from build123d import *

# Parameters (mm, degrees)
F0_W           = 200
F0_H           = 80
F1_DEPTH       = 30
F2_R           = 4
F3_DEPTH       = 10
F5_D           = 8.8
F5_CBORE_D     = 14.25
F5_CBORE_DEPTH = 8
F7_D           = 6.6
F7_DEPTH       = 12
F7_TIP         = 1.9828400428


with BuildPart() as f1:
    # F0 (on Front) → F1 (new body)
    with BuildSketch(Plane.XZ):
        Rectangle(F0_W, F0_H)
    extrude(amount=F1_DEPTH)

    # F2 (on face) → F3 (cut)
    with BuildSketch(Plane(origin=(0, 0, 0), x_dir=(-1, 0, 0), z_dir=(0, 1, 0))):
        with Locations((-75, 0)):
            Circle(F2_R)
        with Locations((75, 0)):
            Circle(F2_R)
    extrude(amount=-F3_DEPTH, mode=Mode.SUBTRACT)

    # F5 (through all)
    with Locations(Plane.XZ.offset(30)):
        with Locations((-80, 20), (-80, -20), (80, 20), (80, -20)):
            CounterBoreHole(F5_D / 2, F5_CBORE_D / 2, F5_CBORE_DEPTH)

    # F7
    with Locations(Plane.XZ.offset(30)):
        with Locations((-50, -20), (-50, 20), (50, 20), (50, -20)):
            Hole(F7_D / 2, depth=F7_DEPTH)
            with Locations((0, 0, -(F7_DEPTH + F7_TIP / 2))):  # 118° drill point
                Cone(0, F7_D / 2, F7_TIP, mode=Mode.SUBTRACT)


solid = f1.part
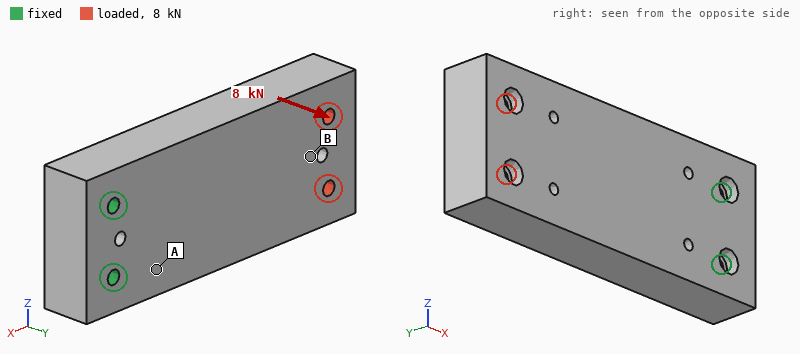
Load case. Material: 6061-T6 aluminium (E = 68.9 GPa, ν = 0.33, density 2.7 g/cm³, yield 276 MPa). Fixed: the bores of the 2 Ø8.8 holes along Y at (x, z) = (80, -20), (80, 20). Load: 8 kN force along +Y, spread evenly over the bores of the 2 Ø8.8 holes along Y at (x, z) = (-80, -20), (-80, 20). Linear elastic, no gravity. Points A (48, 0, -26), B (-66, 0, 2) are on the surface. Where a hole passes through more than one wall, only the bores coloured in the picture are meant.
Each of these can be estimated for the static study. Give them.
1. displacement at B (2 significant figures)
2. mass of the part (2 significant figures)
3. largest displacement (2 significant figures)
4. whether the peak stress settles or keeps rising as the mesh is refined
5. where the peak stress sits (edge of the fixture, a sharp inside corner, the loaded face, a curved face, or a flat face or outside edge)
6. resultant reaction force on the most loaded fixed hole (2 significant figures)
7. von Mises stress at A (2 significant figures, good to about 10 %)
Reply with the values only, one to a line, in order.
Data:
1.0 mm
1.3 kg
1.4 mm
keeps rising
edge of the fixture
4.4 kN
87 MPa
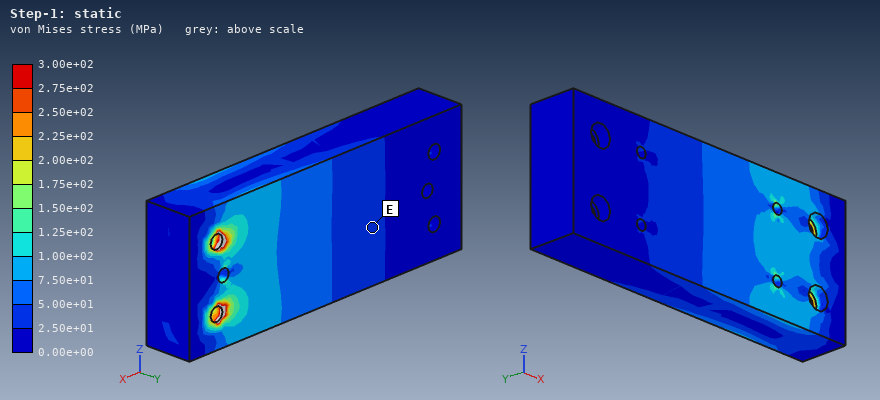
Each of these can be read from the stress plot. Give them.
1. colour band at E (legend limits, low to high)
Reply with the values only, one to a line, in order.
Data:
2.50e+01 to 5.00e+01 MPa
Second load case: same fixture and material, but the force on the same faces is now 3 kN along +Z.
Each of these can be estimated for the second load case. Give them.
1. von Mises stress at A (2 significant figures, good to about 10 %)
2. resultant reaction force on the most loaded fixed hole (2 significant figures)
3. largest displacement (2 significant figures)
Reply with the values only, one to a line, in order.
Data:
9.6 MPa
11 kN
92 µm
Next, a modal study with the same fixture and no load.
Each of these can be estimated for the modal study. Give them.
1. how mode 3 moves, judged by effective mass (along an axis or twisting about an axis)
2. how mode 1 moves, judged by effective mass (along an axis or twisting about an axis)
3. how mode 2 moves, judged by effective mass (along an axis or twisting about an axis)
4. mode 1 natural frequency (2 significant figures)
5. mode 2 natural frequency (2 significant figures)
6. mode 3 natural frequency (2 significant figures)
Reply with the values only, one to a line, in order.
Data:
twisting about X
along Y
along Z
650 Hz
1500 Hz
2700 Hz
